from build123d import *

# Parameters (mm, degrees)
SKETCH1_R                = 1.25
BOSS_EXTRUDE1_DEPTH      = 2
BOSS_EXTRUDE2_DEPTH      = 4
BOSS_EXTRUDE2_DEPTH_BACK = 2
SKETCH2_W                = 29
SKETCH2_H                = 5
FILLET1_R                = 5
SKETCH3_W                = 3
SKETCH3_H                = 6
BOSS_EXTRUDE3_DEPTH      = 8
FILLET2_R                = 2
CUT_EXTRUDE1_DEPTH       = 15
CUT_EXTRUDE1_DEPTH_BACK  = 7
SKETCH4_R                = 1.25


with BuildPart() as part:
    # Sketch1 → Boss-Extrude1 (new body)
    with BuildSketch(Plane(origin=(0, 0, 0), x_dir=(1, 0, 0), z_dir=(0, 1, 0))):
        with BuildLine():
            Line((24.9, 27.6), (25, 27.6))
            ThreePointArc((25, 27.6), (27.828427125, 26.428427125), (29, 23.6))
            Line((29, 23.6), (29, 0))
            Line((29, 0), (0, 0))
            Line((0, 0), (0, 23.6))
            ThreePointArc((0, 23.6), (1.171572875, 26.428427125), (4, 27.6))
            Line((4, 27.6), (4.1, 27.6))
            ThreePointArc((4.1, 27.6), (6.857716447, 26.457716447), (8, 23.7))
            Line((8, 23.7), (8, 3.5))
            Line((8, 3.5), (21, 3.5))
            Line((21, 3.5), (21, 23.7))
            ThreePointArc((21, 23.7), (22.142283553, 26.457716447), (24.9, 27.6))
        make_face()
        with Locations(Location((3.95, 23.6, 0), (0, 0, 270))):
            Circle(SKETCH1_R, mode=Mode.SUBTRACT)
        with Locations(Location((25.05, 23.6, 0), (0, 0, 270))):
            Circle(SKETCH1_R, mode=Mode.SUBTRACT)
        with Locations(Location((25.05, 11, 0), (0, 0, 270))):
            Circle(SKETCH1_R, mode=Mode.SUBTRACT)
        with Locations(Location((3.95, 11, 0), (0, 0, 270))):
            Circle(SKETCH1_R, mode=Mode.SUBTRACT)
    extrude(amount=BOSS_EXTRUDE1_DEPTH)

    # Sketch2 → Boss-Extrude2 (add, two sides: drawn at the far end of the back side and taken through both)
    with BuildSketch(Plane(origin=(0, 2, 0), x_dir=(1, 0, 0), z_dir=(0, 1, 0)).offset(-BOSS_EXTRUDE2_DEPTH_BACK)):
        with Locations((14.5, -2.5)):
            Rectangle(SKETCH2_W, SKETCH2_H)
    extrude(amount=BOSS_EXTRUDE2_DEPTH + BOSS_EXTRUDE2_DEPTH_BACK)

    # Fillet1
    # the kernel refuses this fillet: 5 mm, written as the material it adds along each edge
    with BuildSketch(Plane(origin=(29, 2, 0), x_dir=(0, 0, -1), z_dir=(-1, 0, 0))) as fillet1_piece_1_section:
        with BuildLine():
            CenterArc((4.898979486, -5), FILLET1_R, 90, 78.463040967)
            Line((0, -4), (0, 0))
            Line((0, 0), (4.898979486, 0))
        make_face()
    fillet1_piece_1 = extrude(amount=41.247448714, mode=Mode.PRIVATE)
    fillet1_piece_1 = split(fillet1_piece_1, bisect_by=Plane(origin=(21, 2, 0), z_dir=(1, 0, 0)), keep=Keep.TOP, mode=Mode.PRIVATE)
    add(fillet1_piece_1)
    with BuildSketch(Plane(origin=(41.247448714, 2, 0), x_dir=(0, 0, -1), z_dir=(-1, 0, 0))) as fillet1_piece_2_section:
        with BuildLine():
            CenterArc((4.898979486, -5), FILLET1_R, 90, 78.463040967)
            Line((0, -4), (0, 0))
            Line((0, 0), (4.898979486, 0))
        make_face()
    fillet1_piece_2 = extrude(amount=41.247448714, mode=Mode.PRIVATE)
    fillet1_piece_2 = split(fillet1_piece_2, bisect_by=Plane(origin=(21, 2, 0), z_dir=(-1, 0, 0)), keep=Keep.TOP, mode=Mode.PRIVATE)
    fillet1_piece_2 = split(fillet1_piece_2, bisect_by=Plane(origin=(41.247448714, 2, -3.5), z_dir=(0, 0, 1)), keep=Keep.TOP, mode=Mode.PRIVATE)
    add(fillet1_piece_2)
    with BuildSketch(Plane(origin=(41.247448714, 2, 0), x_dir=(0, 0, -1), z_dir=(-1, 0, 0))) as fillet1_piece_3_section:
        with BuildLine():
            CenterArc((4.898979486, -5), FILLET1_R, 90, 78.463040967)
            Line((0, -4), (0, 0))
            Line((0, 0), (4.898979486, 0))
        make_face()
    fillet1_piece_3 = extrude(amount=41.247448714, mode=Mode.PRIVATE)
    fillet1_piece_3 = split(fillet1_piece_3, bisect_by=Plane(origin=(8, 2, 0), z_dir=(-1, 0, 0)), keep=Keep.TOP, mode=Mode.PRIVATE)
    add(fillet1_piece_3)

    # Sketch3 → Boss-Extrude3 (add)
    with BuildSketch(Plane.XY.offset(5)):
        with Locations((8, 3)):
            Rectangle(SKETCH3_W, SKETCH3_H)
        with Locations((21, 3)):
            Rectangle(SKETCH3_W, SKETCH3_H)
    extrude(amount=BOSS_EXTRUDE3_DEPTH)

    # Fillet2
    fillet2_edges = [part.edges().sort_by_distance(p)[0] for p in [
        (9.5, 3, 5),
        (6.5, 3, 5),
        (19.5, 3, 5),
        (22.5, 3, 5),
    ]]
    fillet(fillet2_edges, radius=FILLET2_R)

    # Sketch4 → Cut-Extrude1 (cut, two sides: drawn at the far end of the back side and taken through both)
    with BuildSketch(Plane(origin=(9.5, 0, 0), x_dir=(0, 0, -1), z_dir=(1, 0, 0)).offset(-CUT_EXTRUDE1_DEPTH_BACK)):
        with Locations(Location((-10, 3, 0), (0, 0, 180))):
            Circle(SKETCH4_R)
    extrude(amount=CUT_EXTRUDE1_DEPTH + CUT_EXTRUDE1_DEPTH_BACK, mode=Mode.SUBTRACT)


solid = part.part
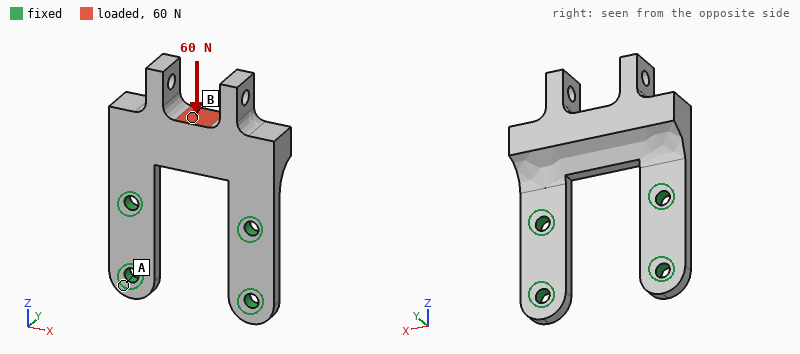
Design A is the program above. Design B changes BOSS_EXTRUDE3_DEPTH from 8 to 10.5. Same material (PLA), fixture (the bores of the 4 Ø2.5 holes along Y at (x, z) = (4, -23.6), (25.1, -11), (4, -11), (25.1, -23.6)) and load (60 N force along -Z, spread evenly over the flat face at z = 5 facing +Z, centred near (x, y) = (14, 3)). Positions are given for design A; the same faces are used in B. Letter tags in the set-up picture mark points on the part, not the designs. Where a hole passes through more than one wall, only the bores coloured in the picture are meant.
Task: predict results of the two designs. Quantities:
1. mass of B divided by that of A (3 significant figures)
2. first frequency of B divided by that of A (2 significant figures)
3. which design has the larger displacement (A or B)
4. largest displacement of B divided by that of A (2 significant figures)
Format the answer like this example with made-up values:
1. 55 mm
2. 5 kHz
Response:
1. 1.04
2. 0.89
3. B
4. 1.1
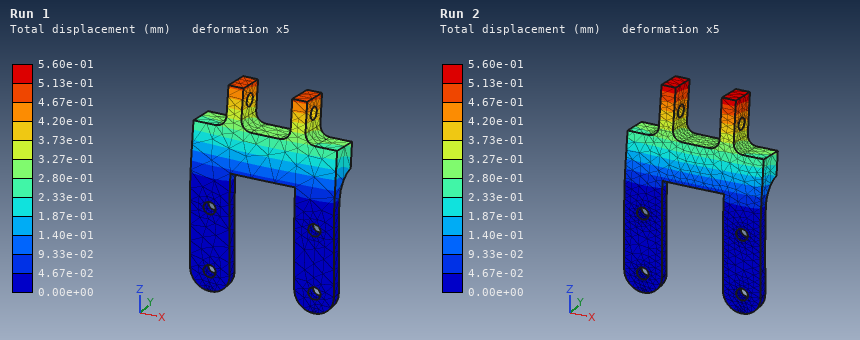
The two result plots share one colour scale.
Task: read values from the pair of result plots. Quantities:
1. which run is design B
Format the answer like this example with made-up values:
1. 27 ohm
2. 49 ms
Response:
1. Run 2
